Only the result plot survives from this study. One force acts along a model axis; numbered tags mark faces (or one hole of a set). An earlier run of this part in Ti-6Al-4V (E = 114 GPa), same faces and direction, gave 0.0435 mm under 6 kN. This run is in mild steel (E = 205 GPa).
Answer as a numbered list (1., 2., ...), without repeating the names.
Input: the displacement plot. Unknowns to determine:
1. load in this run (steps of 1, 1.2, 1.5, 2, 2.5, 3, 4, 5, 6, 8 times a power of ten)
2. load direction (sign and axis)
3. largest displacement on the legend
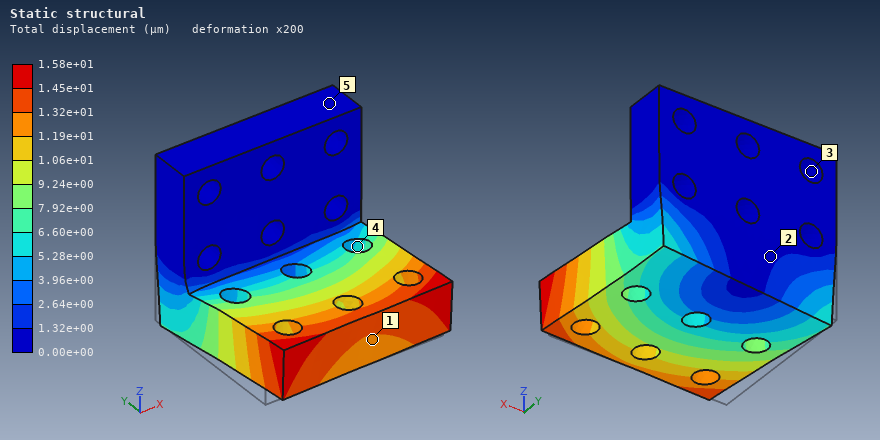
1. 4 kN
2. +X
3. 1.58e+01 µm
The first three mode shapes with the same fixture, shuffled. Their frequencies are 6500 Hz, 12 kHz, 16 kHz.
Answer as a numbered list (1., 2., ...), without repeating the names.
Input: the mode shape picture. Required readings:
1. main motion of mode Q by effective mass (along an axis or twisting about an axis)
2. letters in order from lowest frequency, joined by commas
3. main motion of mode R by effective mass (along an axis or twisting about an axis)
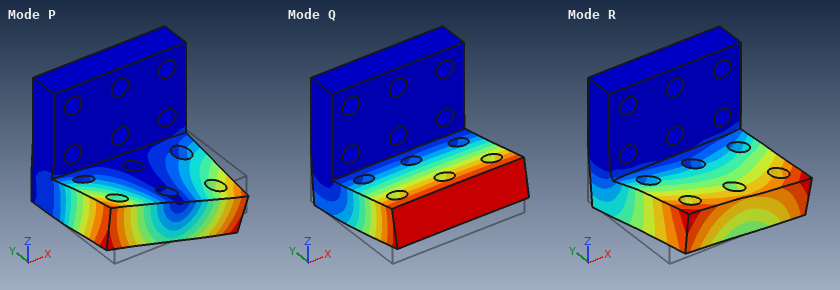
1. along Z
2. Q, R, P
3. along X
